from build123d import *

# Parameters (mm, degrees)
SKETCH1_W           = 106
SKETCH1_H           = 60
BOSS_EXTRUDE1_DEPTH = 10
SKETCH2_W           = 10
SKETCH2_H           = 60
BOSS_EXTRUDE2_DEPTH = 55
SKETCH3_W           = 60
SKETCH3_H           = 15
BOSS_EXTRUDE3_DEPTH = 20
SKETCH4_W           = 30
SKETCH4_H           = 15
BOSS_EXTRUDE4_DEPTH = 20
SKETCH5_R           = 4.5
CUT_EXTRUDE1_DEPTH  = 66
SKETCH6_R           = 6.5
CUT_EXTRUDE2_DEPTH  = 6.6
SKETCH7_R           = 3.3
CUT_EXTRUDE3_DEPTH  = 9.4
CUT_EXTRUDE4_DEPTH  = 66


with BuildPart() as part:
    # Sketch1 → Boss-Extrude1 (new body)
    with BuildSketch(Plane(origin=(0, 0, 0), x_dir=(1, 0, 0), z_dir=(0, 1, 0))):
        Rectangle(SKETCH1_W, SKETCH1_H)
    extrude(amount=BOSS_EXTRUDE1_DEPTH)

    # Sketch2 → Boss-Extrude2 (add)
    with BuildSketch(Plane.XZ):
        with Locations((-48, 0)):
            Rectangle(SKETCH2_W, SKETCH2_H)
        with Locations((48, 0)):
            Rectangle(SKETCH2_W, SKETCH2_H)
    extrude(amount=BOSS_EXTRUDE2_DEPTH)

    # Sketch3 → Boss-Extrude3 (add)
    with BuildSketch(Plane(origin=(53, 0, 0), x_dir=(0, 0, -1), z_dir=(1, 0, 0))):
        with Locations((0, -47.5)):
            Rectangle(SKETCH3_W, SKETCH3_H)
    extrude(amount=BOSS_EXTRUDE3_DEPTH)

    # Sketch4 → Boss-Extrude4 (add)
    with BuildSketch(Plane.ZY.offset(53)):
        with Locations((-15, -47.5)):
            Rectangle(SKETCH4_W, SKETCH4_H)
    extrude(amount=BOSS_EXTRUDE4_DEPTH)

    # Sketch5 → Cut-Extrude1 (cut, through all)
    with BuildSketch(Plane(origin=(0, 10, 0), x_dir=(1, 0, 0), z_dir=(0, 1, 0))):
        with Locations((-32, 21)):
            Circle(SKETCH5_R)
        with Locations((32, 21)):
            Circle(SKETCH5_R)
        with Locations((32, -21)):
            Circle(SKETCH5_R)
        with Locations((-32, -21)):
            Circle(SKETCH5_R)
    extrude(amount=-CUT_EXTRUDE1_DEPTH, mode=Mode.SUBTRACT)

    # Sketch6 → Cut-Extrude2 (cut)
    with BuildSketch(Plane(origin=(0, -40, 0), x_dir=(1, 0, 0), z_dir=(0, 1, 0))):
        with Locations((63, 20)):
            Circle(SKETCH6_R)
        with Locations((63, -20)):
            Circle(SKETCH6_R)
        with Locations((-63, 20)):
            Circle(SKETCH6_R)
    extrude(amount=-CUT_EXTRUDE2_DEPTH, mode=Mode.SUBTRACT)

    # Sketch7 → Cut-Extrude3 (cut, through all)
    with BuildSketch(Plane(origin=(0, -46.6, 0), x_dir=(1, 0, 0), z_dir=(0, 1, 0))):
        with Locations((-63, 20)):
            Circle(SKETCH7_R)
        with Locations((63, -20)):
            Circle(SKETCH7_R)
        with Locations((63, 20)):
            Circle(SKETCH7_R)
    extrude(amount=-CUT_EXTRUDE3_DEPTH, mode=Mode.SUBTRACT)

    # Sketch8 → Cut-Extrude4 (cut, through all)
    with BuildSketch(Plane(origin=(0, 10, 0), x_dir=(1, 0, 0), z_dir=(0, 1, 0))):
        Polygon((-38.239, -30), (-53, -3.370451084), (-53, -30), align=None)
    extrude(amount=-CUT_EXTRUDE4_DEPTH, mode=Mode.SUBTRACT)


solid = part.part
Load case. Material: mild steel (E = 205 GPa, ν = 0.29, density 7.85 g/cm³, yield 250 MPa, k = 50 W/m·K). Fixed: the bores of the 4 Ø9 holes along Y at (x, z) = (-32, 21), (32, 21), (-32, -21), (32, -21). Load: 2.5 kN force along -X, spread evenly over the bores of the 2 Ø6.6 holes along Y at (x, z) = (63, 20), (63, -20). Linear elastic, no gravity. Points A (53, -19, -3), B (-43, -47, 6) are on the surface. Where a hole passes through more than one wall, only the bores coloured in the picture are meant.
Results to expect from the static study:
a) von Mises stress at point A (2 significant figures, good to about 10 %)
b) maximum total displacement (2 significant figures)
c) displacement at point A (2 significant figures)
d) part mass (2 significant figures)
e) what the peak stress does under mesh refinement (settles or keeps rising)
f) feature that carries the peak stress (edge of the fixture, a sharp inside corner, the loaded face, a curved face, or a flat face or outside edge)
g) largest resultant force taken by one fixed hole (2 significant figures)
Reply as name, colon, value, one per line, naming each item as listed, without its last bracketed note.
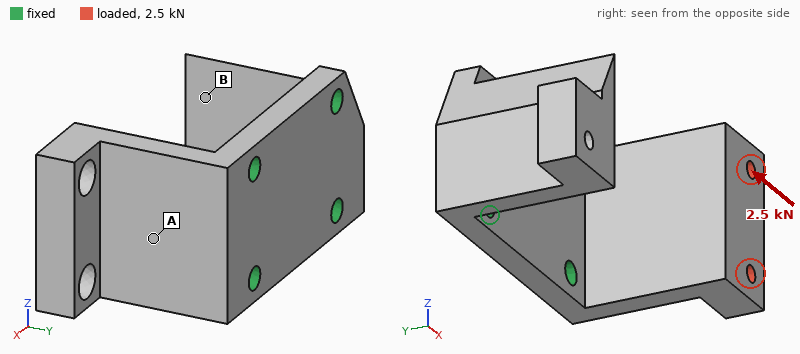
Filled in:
von Mises stress at point A: 69 MPa
maximum total displacement: 0.28 mm
displacement at point A: 0.079 mm
part mass: 1.1 kg
what the peak stress does under mesh refinement: keeps rising
feature that carries the peak stress: edge of the fixture
largest resultant force taken by one fixed hole: 1.2 kN
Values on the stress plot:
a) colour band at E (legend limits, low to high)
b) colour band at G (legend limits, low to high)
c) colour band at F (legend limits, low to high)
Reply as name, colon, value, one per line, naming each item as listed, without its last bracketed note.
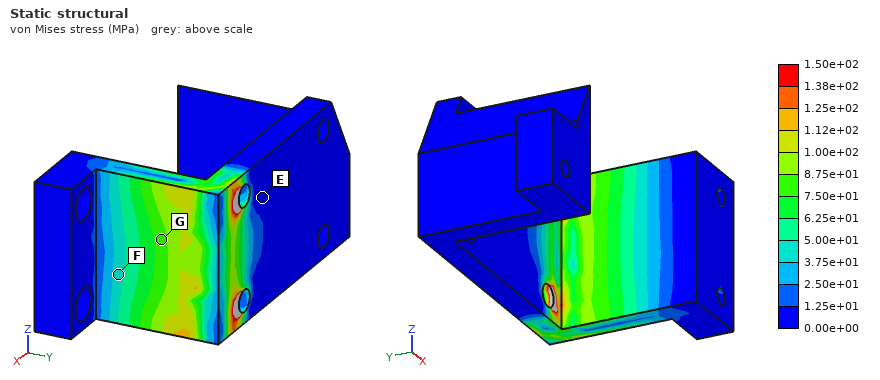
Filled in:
colour band at E: 0.00e+00 to 1.25e+01 MPa
colour band at G: 7.50e+01 to 8.75e+01 MPa
colour band at F: 3.75e+01 to 5.00e+01 MPa
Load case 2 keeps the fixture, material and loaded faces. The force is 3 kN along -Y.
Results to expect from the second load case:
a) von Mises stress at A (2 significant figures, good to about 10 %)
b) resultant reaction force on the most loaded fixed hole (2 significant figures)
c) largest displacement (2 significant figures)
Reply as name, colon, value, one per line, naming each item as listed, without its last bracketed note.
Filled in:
von Mises stress at A: 44 MPa
resultant reaction force on the most loaded fixed hole: 1.6 kN
largest displacement: 0.15 mm
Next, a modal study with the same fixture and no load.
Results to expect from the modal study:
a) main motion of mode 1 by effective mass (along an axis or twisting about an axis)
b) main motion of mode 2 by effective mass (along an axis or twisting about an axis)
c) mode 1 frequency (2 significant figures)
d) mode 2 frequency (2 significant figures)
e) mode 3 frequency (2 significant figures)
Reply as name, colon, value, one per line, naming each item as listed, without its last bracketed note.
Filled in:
main motion of mode 1 by effective mass: along X
main motion of mode 2 by effective mass: along X
mode 1 frequency: 1100 Hz
mode 2 frequency: 1200 Hz
mode 3 frequency: 3300 Hz
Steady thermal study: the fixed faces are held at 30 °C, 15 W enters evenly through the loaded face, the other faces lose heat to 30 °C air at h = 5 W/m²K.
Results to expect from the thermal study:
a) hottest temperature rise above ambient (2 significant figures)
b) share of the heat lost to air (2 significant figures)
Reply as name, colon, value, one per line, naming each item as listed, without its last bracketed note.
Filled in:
hottest temperature rise above ambient: 37 K
share of the heat lost to air: 9.9 %
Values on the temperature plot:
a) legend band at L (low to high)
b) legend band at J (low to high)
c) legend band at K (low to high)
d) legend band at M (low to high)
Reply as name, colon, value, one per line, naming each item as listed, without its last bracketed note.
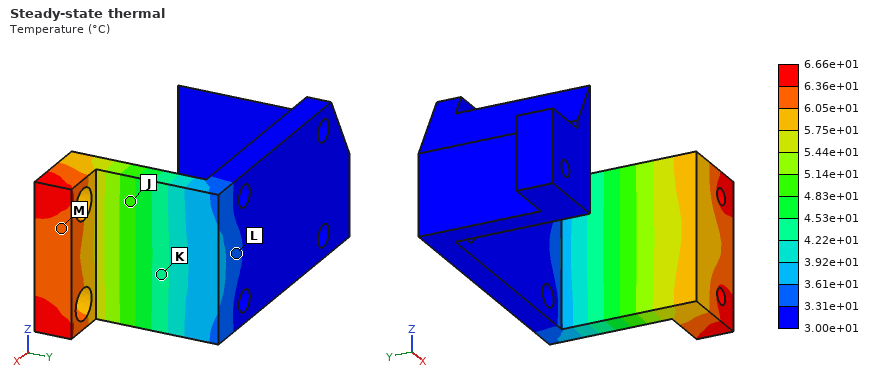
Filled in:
legend band at L: 3.31e+01 to 3.61e+01 °C
legend band at J: 4.83e+01 to 5.14e+01 °C
legend band at K: 4.22e+01 to 4.53e+01 °C
legend band at M: 6.05e+01 to 6.36e+01 °C
